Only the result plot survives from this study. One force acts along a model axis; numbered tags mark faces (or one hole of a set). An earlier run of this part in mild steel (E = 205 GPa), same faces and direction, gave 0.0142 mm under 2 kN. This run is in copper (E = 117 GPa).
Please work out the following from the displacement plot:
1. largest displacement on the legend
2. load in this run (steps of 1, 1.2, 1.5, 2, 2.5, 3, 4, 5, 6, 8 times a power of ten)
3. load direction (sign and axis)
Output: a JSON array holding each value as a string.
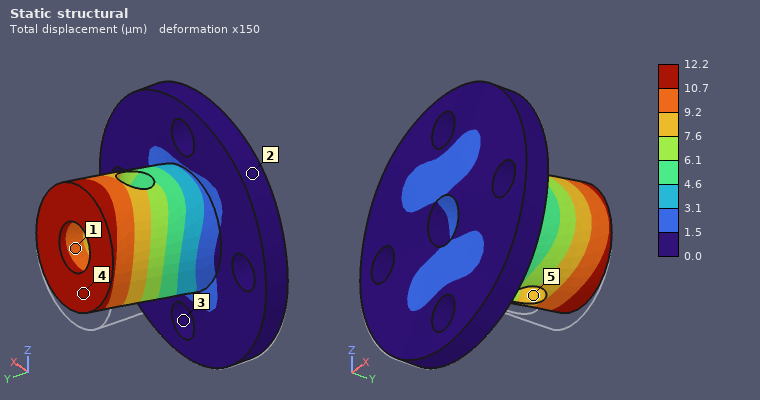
["12.2 µm", "1 kN", "+Z"]
